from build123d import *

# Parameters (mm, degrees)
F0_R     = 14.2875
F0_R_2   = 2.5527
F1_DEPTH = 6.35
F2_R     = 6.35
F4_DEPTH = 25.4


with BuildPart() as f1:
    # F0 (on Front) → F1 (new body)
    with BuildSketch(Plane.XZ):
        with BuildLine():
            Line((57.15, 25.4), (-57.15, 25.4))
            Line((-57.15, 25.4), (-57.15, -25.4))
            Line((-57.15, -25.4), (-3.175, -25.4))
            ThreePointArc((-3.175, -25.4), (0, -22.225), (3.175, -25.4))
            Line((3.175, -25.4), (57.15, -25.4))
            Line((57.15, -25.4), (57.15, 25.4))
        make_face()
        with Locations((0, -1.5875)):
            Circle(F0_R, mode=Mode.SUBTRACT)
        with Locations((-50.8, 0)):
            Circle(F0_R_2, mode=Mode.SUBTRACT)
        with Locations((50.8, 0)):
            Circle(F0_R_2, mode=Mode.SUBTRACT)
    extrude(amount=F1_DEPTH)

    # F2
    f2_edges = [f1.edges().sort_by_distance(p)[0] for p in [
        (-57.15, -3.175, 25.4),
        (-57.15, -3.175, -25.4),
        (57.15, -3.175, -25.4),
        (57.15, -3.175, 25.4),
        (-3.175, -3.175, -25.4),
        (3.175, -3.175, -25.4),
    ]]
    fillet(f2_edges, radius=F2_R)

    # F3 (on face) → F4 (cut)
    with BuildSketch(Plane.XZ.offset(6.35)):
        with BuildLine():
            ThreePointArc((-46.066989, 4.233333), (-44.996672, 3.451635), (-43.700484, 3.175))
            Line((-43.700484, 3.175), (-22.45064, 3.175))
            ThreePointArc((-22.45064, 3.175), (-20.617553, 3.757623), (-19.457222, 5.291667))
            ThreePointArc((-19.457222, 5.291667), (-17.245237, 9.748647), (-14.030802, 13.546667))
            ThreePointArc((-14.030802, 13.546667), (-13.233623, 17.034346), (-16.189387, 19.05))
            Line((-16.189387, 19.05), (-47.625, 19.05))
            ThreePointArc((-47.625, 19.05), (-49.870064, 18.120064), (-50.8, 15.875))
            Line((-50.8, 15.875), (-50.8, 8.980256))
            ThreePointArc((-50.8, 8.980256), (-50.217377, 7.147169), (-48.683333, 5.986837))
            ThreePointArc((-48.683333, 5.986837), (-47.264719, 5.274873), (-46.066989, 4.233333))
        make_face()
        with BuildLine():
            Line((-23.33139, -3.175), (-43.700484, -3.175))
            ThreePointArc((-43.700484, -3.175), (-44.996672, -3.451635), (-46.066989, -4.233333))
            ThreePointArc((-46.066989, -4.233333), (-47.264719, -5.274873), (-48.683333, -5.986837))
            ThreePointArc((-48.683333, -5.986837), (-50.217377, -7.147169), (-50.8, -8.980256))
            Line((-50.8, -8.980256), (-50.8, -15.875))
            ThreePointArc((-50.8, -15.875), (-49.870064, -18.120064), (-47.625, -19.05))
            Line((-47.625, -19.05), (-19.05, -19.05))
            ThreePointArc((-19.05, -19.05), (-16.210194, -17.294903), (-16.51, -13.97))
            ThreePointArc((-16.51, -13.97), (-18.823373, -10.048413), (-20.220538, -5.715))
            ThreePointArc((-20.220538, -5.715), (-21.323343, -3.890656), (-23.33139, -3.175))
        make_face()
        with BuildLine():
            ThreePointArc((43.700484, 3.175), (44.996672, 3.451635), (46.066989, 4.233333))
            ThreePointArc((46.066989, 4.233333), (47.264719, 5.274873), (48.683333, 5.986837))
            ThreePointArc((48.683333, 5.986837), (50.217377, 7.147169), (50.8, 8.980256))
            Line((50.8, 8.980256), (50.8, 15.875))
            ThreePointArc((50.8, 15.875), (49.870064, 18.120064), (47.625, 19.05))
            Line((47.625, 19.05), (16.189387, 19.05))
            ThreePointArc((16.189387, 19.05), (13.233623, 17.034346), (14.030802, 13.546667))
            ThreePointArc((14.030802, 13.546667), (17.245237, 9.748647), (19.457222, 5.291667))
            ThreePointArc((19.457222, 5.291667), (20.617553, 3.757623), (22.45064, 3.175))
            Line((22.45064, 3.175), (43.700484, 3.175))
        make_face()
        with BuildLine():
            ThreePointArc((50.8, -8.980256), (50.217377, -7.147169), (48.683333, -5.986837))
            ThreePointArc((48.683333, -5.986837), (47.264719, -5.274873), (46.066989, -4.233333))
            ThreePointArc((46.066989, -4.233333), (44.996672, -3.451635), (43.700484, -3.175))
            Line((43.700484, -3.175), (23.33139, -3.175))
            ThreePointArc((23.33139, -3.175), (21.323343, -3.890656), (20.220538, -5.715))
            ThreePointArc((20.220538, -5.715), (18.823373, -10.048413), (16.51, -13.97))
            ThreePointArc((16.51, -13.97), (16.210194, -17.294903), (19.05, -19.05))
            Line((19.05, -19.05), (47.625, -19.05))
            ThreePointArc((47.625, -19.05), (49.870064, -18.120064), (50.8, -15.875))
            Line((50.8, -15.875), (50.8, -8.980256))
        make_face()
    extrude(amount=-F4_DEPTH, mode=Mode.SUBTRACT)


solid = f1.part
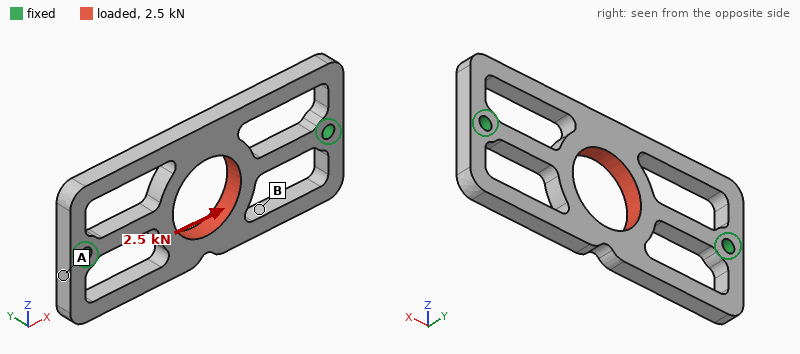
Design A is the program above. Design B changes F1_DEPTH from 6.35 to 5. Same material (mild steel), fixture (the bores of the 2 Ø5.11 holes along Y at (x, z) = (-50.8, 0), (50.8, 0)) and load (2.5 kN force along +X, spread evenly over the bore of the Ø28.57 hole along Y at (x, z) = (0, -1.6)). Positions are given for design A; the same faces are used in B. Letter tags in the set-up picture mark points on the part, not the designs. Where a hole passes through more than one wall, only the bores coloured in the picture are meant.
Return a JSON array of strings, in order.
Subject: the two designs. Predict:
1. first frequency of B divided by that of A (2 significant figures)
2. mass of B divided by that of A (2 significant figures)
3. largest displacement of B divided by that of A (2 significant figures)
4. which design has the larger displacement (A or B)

["0.82", "0.79", "1.3", "B"]
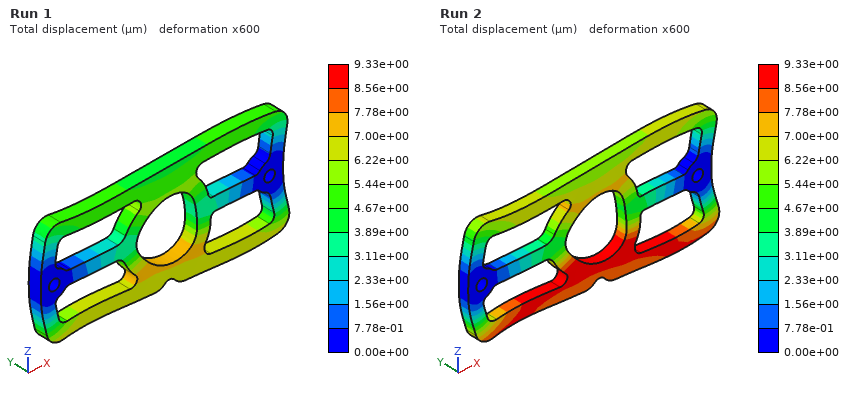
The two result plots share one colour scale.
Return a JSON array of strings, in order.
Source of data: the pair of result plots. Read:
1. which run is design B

["Run 2"]
